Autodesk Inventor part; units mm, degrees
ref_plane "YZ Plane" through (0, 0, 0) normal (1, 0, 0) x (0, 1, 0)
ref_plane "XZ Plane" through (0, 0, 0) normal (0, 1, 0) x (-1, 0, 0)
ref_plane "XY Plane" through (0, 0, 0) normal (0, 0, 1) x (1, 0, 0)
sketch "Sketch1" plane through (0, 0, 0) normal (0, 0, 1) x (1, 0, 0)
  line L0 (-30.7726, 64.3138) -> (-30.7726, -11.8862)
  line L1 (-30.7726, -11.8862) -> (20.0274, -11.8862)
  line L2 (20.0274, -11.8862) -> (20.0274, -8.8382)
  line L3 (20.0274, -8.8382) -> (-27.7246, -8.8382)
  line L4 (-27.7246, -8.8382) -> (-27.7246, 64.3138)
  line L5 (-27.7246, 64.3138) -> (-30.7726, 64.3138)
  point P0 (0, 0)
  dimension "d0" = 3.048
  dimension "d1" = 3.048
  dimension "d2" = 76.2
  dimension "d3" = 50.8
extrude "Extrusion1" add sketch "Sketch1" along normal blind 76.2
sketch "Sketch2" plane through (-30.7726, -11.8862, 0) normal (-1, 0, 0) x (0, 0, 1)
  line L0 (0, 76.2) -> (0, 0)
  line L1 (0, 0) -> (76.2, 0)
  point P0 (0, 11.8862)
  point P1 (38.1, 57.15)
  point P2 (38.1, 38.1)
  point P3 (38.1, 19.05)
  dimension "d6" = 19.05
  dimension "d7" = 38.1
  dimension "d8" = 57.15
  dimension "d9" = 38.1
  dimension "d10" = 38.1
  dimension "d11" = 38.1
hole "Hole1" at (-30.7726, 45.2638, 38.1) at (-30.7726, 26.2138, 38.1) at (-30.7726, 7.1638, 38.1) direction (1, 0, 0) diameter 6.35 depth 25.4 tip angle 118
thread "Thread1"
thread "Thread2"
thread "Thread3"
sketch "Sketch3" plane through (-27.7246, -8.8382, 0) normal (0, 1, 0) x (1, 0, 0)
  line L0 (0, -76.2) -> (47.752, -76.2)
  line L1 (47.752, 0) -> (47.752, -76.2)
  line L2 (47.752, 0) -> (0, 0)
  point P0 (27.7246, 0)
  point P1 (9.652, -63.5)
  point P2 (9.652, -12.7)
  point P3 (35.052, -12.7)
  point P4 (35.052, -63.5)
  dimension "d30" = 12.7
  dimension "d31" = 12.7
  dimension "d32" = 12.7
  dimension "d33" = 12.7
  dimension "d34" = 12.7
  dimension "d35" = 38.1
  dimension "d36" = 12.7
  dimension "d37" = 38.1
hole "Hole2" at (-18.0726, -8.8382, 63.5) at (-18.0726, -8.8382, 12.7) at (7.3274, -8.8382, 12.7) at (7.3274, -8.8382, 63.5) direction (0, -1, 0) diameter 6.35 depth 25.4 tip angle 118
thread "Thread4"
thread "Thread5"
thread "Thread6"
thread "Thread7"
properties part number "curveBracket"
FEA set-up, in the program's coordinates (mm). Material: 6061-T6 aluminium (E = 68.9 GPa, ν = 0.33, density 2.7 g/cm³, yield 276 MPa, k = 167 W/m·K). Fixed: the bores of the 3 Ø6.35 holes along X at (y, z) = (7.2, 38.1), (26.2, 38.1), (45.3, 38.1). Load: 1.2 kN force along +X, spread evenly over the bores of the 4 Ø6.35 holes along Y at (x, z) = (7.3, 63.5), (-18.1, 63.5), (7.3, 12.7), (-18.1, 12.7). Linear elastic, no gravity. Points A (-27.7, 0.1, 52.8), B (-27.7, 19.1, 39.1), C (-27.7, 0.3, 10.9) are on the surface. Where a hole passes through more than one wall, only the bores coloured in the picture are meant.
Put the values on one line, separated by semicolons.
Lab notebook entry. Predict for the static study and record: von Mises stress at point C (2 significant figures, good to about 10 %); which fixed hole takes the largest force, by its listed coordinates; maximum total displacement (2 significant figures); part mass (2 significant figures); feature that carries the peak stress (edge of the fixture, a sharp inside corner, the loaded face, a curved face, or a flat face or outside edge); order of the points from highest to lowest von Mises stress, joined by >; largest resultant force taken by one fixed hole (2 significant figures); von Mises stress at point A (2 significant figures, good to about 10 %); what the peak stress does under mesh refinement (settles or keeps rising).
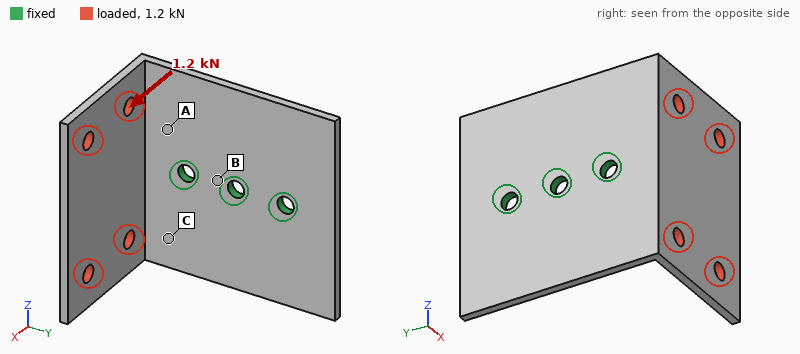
55 MPa; (7.2, 38.1); 0.94 mm; 76 g; edge of the fixture; A > C > B; 1.5 kN; 93 MPa; keeps rising
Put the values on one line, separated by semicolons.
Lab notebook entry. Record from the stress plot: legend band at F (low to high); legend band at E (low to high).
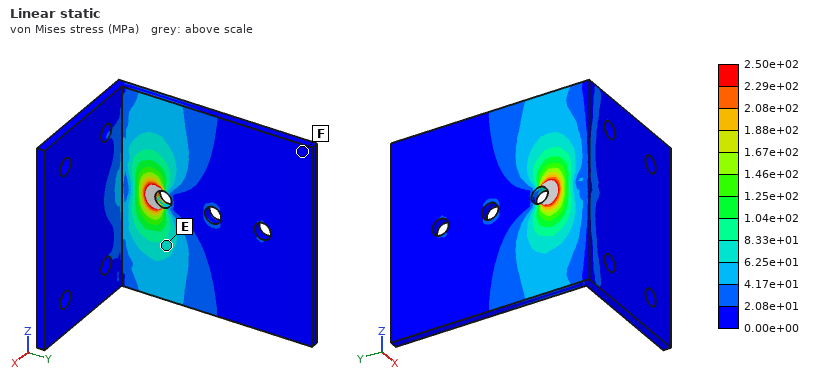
0.00e+00 to 2.08e+01 MPa; 6.25e+01 to 8.33e+01 MPa
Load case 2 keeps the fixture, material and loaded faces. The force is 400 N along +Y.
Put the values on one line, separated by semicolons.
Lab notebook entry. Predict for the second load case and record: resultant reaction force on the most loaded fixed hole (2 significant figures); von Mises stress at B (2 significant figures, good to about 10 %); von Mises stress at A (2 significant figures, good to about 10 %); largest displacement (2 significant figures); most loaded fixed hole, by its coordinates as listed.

300 N; 20 MPa; 72 MPa; 1.2 mm; (7.2, 38.1)
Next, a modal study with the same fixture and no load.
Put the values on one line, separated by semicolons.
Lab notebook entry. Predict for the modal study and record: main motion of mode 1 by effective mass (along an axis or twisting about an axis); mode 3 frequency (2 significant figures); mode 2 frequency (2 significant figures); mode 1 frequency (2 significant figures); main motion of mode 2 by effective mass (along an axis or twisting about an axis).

along Y; 1600 Hz; 800 Hz; 640 Hz; along Z
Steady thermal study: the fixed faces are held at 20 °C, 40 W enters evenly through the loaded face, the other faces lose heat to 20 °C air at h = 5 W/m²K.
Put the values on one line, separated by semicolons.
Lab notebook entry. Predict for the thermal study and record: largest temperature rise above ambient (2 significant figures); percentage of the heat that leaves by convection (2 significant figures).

57 K; 5.6 %
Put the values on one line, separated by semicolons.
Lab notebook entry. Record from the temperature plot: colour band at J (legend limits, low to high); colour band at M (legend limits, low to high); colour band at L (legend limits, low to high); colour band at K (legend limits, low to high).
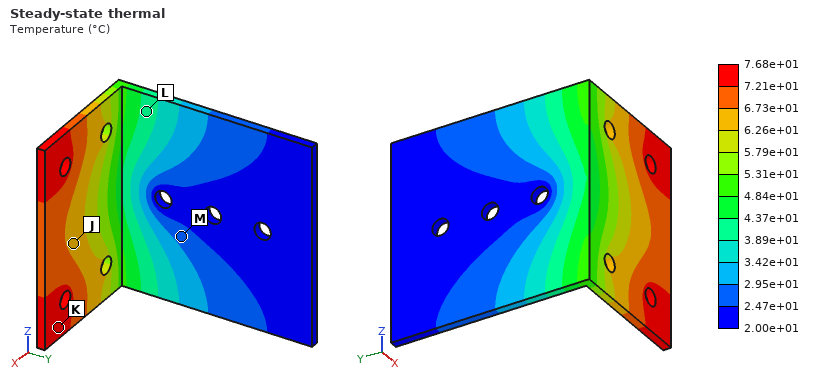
6.26e+01 to 6.73e+01 °C; 2.47e+01 to 2.95e+01 °C; 3.89e+01 to 4.37e+01 °C; 7.21e+01 to 7.68e+01 °C
